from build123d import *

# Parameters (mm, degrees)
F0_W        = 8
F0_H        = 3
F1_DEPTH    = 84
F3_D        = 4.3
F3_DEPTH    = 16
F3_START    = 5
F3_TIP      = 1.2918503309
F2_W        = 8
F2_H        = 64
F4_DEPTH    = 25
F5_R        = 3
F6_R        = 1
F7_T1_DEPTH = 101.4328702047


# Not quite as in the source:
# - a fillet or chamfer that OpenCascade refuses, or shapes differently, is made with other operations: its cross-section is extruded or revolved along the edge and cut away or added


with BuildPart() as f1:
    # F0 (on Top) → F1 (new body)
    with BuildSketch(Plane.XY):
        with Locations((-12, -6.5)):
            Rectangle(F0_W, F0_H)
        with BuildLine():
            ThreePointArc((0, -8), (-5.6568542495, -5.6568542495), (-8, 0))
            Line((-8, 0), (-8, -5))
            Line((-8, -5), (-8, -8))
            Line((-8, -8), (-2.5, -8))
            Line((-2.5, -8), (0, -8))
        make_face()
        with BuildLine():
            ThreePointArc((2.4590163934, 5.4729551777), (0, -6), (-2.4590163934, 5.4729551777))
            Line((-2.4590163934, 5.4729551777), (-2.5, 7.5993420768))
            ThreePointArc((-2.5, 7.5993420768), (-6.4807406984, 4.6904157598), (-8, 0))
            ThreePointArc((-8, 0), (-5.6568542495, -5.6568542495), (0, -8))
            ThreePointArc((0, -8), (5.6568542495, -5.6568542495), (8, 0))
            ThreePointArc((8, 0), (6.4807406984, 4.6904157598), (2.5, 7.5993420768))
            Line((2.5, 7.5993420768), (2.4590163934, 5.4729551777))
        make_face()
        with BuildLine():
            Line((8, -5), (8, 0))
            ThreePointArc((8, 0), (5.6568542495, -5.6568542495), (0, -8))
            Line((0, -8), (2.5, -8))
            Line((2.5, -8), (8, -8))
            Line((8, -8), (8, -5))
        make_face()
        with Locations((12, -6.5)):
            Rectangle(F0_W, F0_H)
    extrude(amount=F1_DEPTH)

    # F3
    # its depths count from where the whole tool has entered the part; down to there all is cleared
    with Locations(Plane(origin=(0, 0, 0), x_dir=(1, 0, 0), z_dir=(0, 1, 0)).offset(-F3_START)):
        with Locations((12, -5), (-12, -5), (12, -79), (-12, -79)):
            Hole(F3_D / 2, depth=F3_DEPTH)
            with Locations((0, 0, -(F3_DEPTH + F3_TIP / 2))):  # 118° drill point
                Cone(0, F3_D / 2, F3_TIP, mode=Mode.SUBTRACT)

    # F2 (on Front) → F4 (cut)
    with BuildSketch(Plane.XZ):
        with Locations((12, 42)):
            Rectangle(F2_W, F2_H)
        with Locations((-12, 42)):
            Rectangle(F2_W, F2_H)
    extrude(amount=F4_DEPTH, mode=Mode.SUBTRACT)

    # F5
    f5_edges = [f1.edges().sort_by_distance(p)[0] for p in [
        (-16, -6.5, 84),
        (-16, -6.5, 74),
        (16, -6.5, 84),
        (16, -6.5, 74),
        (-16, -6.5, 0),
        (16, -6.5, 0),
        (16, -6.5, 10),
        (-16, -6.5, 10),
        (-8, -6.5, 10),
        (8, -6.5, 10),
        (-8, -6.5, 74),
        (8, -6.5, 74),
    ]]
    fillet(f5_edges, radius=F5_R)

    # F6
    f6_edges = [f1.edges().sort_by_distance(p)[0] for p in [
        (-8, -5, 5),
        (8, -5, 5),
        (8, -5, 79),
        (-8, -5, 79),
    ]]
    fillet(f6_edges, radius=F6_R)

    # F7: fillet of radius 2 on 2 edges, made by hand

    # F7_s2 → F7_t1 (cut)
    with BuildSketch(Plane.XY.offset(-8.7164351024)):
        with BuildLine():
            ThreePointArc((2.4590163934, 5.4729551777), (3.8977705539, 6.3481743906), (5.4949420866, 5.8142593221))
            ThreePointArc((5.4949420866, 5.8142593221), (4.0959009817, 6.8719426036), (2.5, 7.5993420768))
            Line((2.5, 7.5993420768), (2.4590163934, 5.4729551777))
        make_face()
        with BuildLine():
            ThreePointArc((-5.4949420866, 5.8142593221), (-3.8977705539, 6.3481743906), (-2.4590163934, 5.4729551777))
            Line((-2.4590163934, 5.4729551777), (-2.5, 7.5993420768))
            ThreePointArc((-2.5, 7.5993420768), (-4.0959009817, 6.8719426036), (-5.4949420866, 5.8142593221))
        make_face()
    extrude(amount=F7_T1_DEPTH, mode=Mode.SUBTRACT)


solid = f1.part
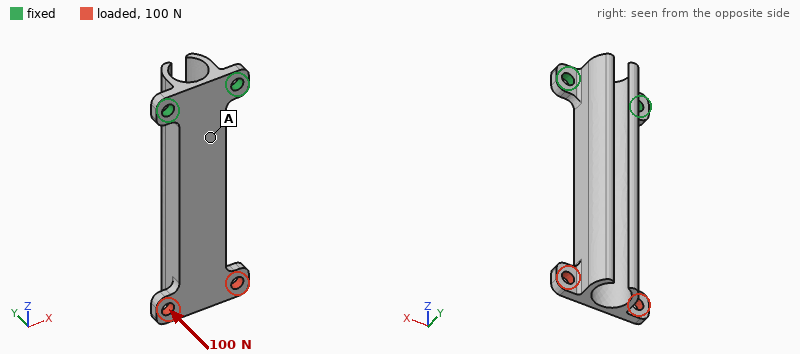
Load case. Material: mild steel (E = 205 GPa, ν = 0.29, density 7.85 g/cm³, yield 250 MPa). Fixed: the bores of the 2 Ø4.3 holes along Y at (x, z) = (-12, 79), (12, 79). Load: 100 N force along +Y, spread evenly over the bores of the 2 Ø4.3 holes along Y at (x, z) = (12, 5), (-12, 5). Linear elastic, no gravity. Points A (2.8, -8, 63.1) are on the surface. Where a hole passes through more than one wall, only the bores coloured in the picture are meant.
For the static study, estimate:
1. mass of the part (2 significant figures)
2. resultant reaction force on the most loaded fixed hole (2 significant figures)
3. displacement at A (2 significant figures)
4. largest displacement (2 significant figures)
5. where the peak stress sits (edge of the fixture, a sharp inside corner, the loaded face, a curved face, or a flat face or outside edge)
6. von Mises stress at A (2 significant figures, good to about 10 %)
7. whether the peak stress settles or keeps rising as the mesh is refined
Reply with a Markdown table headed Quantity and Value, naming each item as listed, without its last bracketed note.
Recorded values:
| Quantity | Value |
|---|---|
| mass of the part | 73 g |
| resultant reaction force on the most loaded fixed hole | 98 N |
| displacement at A | 0.027 mm |
| largest displacement | 0.16 mm |
| where the peak stress sits | edge of the fixture |
| von Mises stress at A | 17 MPa |
| whether the peak stress settles or keeps rising as the mesh is refined | keeps rising |
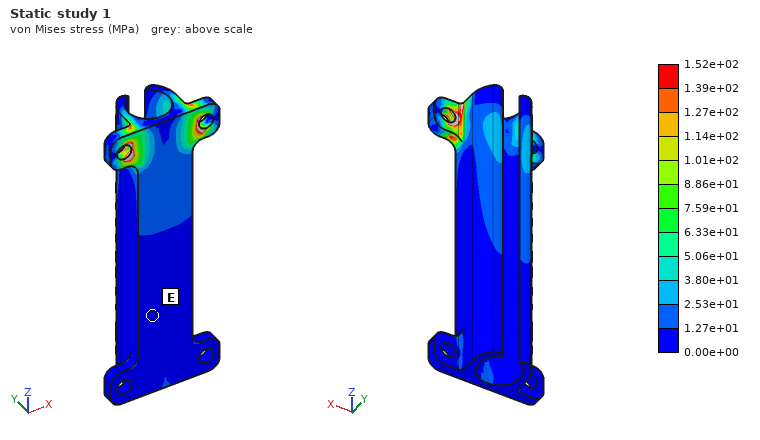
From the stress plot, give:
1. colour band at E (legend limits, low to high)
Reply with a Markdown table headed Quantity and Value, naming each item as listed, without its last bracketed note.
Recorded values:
| Quantity | Value |
|---|---|
| colour band at E | 0.00e+00 to 1.27e+01 MPa |
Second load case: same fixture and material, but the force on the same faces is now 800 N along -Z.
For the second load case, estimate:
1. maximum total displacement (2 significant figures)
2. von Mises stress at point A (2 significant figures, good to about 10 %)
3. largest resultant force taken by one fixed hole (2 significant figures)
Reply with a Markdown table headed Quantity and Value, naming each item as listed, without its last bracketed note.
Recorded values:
| Quantity | Value |
|---|---|
| maximum total displacement | 26 µm |
| von Mises stress at point A | 16 MPa |
| largest resultant force taken by one fixed hole | 420 N |
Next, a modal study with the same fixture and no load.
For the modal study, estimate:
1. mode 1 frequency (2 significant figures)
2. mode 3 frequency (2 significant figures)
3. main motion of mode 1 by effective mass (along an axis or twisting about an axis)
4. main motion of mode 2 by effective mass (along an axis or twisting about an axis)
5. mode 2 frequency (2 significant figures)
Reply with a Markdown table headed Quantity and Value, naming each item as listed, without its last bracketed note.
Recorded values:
| Quantity | Value |
|---|---|
| mode 1 frequency | 810 Hz |
| mode 3 frequency | 2500 Hz |
| main motion of mode 1 by effective mass | along Y |
| main motion of mode 2 by effective mass | along X |
| mode 2 frequency | 1600 Hz |
